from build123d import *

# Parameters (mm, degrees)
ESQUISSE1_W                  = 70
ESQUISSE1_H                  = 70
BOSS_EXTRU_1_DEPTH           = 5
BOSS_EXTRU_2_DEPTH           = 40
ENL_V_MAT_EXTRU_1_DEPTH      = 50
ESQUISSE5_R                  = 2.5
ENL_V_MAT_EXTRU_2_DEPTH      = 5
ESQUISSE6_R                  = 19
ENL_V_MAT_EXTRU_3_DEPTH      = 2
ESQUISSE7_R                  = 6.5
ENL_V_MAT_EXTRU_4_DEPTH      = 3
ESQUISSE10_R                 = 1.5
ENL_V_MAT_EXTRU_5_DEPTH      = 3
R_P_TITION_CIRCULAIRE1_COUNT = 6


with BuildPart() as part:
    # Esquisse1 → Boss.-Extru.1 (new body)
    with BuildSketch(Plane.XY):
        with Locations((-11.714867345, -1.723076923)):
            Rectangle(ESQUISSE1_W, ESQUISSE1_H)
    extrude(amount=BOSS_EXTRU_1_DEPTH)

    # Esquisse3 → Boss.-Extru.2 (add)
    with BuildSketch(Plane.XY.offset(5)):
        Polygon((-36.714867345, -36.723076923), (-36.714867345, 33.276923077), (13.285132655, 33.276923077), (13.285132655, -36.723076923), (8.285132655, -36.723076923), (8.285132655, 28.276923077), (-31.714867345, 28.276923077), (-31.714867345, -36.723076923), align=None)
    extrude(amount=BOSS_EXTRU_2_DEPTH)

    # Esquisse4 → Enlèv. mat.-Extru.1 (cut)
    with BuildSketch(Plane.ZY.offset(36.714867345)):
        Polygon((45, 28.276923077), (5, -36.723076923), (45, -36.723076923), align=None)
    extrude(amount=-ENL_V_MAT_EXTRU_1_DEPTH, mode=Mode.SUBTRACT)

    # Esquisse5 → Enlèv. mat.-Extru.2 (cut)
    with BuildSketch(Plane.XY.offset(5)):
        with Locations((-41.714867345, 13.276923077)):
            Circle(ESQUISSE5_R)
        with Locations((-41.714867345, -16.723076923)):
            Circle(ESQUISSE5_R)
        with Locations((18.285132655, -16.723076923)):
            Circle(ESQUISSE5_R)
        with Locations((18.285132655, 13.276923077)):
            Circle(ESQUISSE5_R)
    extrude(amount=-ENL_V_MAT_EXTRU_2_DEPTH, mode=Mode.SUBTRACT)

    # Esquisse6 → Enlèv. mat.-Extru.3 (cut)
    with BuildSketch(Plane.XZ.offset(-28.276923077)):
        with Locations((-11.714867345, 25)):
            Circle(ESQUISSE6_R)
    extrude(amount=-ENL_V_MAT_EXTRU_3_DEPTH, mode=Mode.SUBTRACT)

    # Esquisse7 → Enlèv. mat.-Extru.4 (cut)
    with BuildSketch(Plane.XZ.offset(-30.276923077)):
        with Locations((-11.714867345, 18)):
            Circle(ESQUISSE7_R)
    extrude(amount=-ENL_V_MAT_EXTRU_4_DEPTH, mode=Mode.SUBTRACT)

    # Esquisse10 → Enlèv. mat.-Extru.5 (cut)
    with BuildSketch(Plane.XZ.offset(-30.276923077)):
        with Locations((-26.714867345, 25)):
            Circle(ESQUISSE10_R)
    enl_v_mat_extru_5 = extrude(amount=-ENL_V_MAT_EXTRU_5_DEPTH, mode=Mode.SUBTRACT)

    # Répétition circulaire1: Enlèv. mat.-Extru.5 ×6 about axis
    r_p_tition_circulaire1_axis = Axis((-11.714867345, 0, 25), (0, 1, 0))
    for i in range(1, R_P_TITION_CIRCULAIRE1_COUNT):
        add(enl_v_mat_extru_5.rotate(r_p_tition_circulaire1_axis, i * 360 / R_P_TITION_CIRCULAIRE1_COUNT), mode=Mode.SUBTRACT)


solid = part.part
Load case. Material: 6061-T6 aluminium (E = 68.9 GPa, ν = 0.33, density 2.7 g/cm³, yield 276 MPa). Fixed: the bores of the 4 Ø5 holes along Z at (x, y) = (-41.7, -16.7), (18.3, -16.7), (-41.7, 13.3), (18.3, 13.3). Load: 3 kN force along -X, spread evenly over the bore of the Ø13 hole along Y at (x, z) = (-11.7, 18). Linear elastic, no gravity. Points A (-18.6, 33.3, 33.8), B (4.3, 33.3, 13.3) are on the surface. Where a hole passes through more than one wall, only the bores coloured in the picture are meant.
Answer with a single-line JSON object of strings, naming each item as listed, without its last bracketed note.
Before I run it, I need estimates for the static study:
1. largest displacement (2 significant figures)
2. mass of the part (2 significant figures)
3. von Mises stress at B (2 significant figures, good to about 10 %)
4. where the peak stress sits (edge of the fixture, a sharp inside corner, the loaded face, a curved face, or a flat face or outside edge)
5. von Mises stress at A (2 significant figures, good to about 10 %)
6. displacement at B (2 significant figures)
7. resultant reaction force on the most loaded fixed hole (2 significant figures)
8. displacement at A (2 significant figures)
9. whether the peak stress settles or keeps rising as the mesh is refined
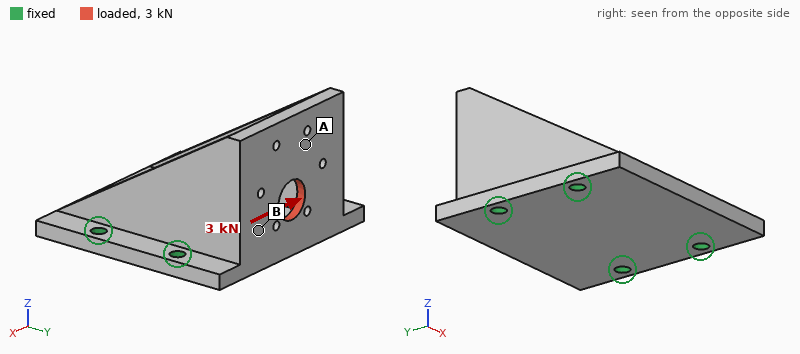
{"largest displacement": "51 µm", "mass of the part": "120 g", "von Mises stress at B": "34 MPa", "where the peak stress sits": "edge of the fixture", "von Mises stress at A": "9.8 MPa", "displacement at B": "23 µm", "resultant reaction force on the most loaded fixed hole": "2.0 kN", "displacement at A": "38 µm", "whether the peak stress settles or keeps rising as the mesh is refined": "keeps rising"}
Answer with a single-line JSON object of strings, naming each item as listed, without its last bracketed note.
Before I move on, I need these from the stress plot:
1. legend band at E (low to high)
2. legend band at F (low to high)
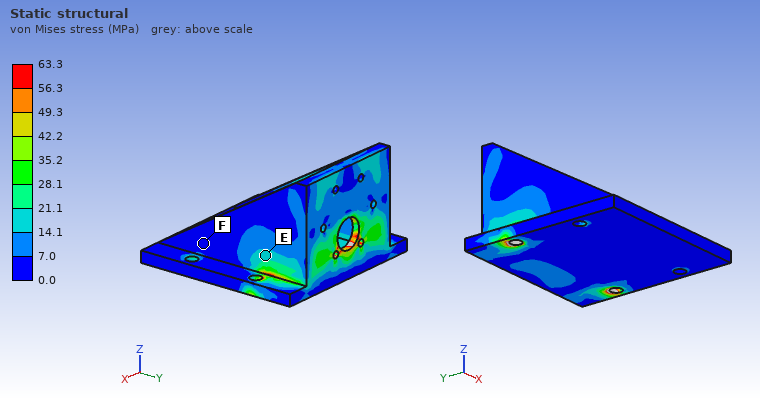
{"legend band at E": "14.1 to 21.1 MPa", "legend band at F": "0.0 to 7.0 MPa"}
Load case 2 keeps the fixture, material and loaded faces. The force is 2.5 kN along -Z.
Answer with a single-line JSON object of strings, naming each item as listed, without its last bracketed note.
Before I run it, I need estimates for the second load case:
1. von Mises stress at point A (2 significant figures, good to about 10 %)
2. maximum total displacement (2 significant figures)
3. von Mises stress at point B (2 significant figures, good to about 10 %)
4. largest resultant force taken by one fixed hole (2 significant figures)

{"von Mises stress at point A": "12 MPa", "maximum total displacement": "68 µm", "von Mises stress at point B": "25 MPa", "largest resultant force taken by one fixed hole": "1.9 kN"}
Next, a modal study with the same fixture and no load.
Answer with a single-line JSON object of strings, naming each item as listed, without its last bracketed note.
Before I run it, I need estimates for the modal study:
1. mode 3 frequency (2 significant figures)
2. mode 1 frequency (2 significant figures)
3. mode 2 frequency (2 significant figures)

{"mode 3 frequency": "5800 Hz", "mode 1 frequency": "5100 Hz", "mode 2 frequency": "5800 Hz"}
